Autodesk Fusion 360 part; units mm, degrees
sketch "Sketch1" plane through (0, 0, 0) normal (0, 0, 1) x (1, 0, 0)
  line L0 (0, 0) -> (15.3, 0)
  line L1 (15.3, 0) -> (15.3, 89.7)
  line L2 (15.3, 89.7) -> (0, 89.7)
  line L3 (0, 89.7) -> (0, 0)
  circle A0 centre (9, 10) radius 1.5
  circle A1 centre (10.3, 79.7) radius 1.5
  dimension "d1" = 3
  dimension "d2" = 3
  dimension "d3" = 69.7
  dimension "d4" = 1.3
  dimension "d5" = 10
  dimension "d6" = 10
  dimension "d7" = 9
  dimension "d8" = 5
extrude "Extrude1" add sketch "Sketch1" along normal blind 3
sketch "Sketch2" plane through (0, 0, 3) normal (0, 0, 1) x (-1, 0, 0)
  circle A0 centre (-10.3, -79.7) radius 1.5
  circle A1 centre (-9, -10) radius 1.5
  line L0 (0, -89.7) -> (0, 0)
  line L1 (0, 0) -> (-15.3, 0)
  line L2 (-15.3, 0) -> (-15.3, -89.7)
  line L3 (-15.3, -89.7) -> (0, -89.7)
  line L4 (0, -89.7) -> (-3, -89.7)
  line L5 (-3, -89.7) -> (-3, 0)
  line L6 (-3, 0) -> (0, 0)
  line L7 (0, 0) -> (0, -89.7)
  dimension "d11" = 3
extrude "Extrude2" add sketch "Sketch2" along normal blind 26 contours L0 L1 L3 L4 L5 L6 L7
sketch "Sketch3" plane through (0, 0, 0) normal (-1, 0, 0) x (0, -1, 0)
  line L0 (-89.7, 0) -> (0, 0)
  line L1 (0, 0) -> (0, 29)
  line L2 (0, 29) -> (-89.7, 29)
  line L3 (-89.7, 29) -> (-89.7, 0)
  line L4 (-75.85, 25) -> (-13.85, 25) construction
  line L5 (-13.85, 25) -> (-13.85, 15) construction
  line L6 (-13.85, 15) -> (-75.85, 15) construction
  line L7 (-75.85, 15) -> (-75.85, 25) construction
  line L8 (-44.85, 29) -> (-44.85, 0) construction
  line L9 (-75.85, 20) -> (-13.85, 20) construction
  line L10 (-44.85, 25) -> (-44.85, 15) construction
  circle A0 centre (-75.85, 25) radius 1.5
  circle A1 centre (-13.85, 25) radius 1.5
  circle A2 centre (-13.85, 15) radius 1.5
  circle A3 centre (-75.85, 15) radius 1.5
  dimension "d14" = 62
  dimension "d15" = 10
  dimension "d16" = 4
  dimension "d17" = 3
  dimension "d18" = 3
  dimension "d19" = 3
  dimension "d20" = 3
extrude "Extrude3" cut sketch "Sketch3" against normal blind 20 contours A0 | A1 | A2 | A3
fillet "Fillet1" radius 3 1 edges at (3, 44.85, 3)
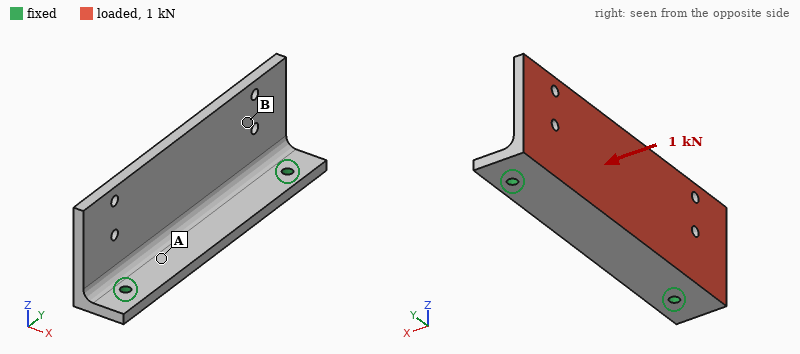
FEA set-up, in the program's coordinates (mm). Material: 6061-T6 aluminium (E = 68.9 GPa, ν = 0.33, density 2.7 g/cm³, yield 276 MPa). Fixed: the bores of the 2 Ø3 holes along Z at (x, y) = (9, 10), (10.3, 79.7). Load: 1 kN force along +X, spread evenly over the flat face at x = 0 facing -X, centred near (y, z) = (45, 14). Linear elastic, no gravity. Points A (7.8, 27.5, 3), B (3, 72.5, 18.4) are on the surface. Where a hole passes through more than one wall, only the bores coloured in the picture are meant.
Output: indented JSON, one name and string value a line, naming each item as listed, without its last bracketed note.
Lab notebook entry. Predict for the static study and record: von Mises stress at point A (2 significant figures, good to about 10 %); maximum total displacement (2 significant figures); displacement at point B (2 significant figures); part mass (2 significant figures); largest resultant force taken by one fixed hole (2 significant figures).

{
  "von Mises stress at point A": "72 MPa",
  "maximum total displacement": "0.59 mm",
  "displacement at point B": "0.31 mm",
  "part mass": "30 g",
  "largest resultant force taken by one fixed hole": "570 N"
}
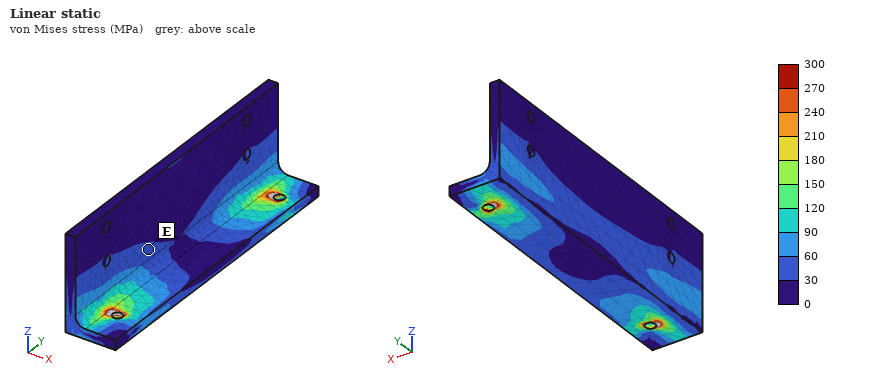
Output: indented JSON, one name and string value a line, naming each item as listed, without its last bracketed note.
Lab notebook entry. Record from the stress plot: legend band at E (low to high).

{
  "legend band at E": "30 to 60 MPa"
}
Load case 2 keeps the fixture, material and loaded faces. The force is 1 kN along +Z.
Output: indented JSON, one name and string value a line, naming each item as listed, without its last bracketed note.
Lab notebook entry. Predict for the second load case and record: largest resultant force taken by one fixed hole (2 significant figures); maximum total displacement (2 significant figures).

{
  "largest resultant force taken by one fixed hole": "510 N",
  "maximum total displacement": "0.24 mm"
}
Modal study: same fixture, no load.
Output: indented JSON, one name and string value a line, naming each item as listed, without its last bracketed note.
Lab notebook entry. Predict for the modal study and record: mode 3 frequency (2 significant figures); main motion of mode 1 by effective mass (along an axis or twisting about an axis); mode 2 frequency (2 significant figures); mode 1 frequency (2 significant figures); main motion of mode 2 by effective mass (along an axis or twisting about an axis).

{
  "mode 3 frequency": "4900 Hz",
  "main motion of mode 1 by effective mass": "along X",
  "mode 2 frequency": "3100 Hz",
  "mode 1 frequency": "1800 Hz",
  "main motion of mode 2 by effective mass": "twisting about Z"
}
